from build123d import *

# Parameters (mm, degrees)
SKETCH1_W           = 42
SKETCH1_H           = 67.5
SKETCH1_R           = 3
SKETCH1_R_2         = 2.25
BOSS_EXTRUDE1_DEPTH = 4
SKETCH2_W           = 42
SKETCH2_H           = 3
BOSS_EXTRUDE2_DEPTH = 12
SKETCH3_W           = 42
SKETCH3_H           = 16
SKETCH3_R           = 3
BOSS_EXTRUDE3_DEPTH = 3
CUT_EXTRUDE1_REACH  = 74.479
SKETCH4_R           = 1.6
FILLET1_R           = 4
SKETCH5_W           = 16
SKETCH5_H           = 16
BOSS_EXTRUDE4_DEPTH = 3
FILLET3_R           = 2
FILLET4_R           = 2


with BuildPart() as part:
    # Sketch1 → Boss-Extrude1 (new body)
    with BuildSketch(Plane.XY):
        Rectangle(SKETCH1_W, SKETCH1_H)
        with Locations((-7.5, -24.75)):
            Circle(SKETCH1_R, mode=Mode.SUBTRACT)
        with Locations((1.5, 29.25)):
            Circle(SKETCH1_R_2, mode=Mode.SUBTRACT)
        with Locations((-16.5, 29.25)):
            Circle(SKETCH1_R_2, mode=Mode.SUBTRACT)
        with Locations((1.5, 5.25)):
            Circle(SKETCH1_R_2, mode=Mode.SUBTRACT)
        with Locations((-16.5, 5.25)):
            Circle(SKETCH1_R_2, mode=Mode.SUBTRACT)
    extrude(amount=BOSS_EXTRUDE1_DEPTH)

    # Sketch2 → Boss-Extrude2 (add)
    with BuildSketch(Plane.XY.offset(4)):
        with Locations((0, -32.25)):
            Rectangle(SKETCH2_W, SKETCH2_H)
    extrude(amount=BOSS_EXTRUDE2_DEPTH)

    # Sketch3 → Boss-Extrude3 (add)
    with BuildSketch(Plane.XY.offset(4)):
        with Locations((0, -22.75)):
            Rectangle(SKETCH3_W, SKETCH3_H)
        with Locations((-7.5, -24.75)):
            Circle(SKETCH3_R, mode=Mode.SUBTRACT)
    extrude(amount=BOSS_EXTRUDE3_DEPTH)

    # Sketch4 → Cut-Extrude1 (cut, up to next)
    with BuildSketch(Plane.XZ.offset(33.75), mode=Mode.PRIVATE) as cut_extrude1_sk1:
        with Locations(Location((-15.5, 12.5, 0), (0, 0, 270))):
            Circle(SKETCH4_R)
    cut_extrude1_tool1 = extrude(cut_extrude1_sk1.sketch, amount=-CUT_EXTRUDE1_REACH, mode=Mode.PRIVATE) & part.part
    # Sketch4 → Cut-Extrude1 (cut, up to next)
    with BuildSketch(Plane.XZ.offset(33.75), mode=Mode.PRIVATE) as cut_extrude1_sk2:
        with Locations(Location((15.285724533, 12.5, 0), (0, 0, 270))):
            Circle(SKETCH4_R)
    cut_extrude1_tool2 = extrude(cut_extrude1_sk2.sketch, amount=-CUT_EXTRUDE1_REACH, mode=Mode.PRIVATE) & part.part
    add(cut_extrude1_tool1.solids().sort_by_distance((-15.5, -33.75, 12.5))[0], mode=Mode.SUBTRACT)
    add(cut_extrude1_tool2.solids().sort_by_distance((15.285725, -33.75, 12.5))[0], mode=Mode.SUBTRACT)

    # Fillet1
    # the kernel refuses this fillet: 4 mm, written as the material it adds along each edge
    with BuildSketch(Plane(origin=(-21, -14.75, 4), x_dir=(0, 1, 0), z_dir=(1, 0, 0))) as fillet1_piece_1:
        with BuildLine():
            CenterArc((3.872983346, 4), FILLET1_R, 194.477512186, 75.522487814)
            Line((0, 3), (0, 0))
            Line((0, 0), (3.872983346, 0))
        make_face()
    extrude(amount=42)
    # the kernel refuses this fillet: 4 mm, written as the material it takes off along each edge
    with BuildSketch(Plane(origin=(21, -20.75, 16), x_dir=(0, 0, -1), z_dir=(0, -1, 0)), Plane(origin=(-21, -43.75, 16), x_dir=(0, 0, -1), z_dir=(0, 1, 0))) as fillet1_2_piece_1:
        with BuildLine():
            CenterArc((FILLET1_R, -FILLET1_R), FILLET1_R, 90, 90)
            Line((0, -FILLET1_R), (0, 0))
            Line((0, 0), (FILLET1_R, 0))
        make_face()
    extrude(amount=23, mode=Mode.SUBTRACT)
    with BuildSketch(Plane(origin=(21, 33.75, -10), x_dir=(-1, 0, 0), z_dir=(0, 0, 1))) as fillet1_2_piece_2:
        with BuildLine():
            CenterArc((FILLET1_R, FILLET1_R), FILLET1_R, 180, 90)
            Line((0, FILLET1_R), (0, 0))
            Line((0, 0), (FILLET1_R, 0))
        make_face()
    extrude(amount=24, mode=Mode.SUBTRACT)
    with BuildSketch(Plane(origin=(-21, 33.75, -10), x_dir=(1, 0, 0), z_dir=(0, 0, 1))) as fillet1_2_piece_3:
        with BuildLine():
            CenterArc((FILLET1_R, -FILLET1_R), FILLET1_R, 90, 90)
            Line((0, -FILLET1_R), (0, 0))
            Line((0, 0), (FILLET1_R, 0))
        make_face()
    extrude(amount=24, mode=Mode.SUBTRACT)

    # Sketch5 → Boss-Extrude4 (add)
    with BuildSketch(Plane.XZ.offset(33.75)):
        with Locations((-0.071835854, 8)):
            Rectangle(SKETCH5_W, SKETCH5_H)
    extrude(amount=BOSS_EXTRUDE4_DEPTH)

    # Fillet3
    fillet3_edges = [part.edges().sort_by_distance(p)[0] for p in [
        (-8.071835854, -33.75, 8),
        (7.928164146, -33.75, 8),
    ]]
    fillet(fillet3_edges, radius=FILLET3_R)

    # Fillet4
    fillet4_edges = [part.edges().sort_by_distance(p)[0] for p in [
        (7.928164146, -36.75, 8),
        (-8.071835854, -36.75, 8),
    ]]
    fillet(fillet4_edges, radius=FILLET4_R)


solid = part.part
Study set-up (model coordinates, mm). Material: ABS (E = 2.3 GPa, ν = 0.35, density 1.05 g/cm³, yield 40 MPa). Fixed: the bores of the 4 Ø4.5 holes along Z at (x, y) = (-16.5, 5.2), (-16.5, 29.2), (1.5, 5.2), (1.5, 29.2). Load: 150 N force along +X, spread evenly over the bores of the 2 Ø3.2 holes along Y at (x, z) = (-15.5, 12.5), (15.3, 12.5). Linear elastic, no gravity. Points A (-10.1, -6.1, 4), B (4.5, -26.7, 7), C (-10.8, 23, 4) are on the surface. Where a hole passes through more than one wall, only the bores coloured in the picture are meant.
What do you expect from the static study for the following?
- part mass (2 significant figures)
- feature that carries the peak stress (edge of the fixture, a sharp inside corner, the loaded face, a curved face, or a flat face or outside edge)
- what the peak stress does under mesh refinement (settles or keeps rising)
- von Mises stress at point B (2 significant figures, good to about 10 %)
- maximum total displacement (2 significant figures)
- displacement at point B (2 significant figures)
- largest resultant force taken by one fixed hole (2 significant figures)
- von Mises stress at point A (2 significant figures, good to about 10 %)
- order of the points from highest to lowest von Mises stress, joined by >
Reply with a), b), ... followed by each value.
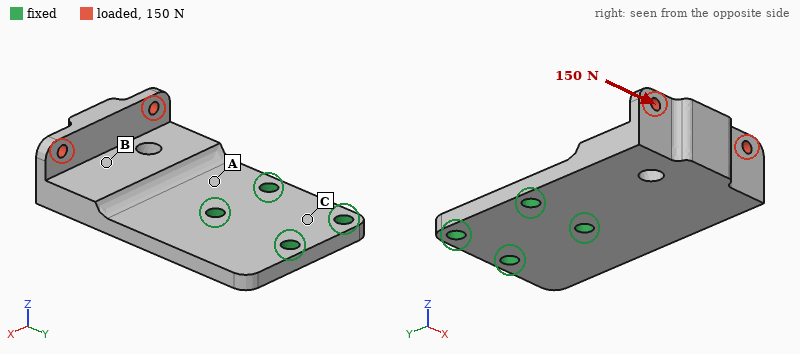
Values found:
a) 16 g
b) edge of the fixture
c) keeps rising
d) 5.4 MPa
e) 0.79 mm
f) 0.29 mm
g) 220 N
h) 9.8 MPa
i) A > B > C
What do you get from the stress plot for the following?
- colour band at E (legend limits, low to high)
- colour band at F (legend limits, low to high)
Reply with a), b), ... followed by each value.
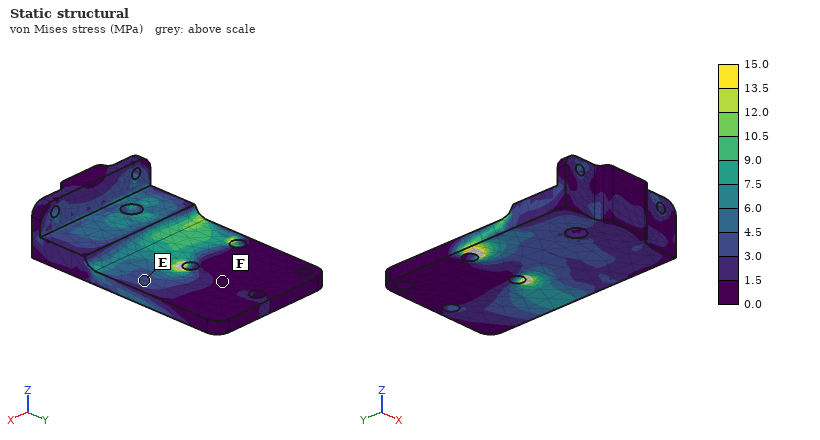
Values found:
a) 3.0 to 4.5 MPa
b) 0.0 to 1.5 MPa
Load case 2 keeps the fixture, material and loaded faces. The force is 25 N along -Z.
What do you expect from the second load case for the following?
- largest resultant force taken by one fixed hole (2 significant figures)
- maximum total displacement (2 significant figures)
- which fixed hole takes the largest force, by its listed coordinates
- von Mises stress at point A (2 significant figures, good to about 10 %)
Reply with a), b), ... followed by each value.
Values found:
a) 29 N
b) 0.95 mm
c) (1.5, 5.2)
d) 5.6 MPa
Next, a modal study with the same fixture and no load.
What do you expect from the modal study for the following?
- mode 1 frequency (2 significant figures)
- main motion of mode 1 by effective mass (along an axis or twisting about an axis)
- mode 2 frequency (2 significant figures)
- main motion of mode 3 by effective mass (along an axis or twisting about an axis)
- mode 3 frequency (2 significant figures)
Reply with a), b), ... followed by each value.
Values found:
a) 390 Hz
b) along Z
c) 1100 Hz
d) along X
e) 2300 Hz
